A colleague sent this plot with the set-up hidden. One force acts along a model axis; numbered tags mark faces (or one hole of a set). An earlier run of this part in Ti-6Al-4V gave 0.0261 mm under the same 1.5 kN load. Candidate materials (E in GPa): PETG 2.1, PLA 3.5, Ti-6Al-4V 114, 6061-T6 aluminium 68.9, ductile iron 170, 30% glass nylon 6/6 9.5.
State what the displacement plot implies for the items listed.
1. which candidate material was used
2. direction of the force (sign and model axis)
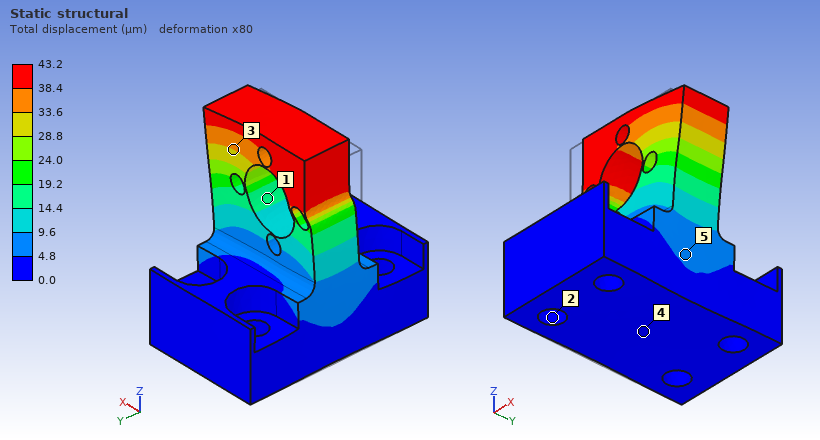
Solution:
6061-T6 aluminium
+X
